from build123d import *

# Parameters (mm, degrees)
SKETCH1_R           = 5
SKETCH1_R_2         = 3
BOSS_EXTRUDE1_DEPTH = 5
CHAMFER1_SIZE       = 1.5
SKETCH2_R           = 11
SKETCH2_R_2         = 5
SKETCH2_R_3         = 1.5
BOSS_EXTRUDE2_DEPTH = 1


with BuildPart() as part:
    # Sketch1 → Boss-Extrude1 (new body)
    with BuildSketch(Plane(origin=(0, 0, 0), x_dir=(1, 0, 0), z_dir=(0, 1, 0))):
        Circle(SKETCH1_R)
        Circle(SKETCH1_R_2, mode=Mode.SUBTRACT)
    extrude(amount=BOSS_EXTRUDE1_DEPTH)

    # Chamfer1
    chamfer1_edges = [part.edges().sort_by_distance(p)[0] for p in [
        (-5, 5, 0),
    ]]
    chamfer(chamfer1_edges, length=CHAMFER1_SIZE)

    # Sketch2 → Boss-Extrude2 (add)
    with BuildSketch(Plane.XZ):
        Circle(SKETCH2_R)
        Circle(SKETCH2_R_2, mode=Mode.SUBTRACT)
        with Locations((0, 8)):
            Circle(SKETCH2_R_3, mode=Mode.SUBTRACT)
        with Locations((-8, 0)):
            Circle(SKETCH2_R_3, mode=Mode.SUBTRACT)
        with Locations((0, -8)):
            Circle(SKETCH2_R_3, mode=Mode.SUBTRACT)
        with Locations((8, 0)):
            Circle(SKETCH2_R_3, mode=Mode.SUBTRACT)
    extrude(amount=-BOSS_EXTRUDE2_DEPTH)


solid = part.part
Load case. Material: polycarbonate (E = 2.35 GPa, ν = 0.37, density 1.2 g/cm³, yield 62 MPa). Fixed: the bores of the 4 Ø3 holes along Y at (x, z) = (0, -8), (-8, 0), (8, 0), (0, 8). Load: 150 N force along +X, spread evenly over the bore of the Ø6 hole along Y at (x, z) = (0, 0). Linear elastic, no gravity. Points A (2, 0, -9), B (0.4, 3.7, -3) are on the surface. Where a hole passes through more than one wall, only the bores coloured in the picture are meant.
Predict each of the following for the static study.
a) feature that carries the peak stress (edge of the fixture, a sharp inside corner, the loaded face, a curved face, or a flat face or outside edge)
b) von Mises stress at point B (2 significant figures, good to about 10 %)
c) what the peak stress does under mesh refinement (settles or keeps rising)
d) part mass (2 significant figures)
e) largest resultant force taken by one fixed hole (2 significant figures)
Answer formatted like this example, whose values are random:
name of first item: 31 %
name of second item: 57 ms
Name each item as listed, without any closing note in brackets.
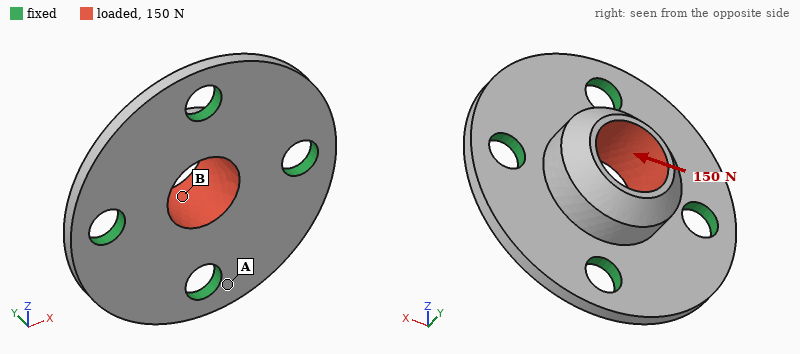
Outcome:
feature that carries the peak stress: edge of the fixture
von Mises stress at point B: 5.9 MPa
what the peak stress does under mesh refinement: keeps rising
part mass: 0.59 g
largest resultant force taken by one fixed hole: 54 N
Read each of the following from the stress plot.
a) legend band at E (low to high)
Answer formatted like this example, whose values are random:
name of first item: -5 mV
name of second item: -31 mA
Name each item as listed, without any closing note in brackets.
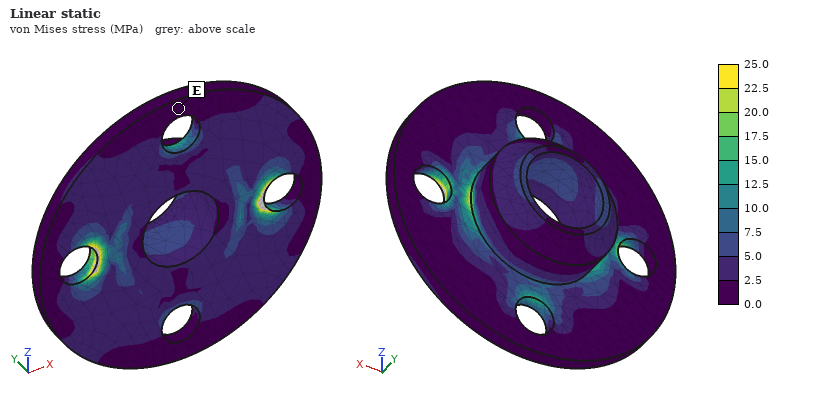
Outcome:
legend band at E: 0.0 to 2.5 MPa
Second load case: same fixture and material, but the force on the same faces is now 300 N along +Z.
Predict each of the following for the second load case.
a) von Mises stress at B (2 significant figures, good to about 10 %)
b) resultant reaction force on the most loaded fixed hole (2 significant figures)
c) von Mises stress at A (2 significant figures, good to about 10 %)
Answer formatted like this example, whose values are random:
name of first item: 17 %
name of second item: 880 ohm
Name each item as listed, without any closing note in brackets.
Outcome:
von Mises stress at B: 9.5 MPa
resultant reaction force on the most loaded fixed hole: 110 N
von Mises stress at A: 7.5 MPa
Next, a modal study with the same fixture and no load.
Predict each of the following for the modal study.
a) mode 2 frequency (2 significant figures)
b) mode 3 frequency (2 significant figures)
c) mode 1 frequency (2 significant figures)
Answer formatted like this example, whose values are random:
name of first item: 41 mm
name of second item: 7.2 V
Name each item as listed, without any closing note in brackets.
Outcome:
mode 2 frequency: 10 kHz
mode 3 frequency: 10 kHz
mode 1 frequency: 10 kHz
